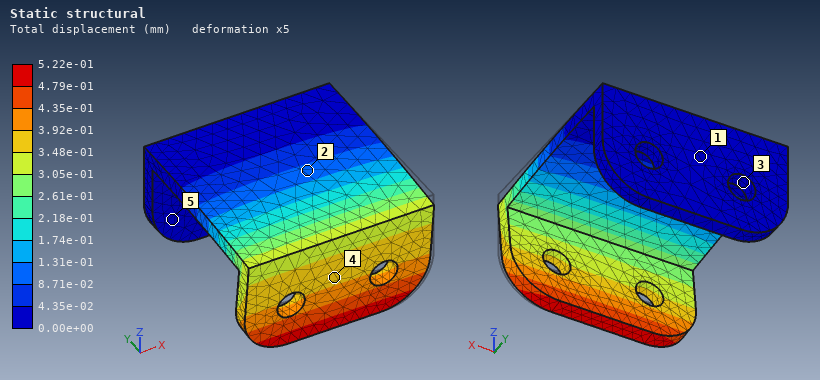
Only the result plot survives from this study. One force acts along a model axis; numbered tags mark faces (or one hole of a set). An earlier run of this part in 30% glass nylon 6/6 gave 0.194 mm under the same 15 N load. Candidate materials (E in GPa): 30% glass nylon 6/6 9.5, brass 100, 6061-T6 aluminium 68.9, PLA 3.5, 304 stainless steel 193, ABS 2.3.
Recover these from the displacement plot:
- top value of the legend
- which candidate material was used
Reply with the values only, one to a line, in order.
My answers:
5.22e-01 mm
PLA
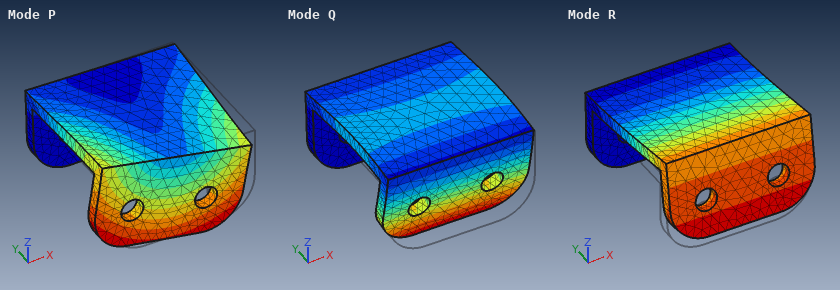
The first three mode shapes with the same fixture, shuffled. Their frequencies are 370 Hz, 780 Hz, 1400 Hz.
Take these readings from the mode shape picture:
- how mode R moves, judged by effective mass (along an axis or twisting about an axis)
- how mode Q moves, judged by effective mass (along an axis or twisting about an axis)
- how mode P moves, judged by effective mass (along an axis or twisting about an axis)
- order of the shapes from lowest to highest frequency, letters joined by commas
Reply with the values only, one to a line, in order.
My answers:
along Z
along Y
along X
R, P, Q
